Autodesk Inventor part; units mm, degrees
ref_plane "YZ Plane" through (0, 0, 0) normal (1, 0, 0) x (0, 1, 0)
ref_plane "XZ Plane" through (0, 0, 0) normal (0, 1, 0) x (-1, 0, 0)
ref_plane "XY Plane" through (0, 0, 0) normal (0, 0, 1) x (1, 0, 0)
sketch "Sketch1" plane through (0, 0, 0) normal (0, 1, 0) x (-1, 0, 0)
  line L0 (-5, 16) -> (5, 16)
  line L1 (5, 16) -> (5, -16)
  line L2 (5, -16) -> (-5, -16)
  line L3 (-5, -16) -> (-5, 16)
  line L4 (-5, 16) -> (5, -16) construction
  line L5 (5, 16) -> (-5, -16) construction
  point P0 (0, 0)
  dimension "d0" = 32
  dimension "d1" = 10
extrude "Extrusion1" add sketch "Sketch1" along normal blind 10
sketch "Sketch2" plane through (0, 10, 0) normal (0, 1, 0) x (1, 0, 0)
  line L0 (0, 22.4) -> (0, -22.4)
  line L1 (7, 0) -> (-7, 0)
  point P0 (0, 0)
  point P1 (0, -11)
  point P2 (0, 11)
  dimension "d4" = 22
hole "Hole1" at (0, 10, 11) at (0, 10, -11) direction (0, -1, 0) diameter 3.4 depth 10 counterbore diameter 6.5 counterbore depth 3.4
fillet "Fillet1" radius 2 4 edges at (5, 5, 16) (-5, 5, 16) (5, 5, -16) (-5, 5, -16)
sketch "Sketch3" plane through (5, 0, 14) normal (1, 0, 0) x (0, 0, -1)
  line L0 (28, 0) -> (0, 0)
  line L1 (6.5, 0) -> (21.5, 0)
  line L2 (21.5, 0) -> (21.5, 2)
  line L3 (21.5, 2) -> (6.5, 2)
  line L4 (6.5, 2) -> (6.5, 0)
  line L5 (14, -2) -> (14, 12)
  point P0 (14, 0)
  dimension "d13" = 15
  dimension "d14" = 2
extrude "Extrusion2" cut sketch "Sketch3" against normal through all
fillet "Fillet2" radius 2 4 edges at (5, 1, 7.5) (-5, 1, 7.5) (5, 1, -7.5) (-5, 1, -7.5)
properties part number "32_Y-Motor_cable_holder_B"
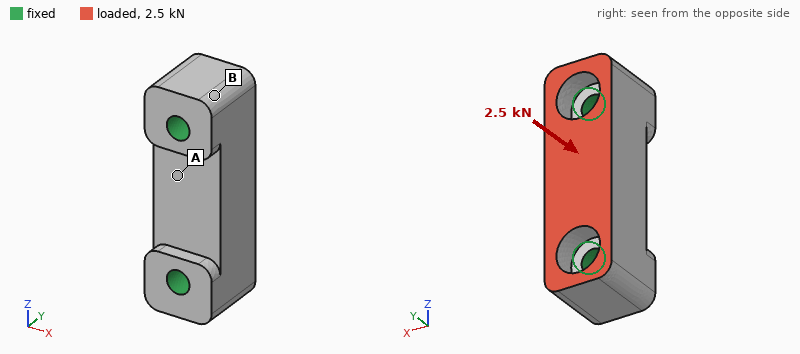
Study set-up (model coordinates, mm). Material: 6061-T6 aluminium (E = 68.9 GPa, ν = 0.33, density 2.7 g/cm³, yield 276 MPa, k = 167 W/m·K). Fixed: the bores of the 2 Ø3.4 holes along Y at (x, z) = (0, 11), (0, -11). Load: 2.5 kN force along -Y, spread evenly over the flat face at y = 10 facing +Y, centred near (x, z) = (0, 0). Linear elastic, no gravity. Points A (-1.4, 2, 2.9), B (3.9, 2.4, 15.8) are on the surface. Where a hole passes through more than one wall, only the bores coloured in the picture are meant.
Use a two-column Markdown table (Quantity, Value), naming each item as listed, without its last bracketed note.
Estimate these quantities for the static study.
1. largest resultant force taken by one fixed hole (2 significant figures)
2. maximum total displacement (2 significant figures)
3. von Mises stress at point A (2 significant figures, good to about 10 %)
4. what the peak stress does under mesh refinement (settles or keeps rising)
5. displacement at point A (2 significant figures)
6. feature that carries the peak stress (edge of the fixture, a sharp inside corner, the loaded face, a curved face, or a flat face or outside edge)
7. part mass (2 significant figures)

| Quantity | Value |
|---|---|
| largest resultant force taken by one fixed hole | 1.3 kN |
| maximum total displacement | 5.9 µm |
| von Mises stress at point A | 14 MPa |
| what the peak stress does under mesh refinement | keeps rising |
| displacement at point A | 4.7 µm |
| feature that carries the peak stress | edge of the fixture |
| part mass | 6.8 g |
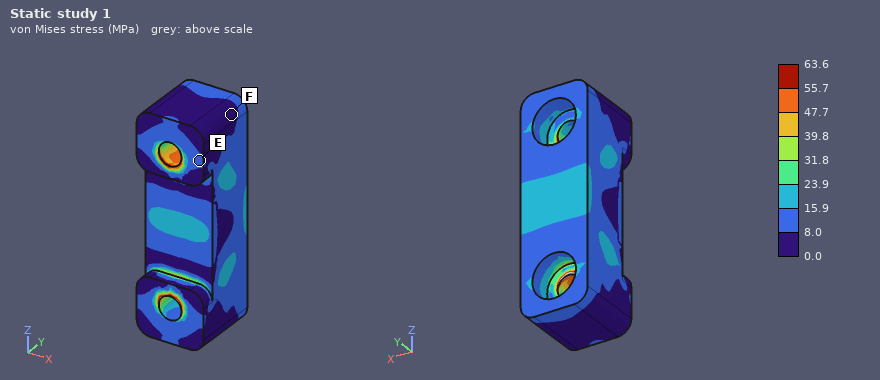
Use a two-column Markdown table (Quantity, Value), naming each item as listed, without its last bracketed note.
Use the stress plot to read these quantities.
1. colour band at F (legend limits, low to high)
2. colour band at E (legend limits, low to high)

| Quantity | Value |
|---|---|
| colour band at F | 0.0 to 8.0 MPa |
| colour band at E | 8.0 to 15.9 MPa |
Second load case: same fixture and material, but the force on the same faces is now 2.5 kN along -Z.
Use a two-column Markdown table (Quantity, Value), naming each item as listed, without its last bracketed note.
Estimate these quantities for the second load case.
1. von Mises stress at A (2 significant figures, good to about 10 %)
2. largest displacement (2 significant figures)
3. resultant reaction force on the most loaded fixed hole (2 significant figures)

| Quantity | Value |
|---|---|
| von Mises stress at A | 8.9 MPa |
| largest displacement | 7.8 µm |
| resultant reaction force on the most loaded fixed hole | 1.4 kN |
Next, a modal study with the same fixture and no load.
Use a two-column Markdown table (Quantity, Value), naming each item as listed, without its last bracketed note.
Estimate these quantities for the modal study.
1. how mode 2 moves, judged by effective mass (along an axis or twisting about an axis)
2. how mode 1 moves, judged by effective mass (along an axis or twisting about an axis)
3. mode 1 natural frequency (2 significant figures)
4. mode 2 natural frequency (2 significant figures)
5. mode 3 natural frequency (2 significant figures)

| Quantity | Value |
|---|---|
| how mode 2 moves, judged by effective mass | along Y |
| how mode 1 moves, judged by effective mass | along X |
| mode 1 natural frequency | 41 kHz |
| mode 2 natural frequency | 50 kHz |
| mode 3 natural frequency | 59 kHz |
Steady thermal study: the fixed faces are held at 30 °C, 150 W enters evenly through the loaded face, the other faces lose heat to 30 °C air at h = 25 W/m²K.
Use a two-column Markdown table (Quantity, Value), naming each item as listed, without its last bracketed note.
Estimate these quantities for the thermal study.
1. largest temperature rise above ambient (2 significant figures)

| Quantity | Value |
|---|---|
| largest temperature rise above ambient | 45 K |
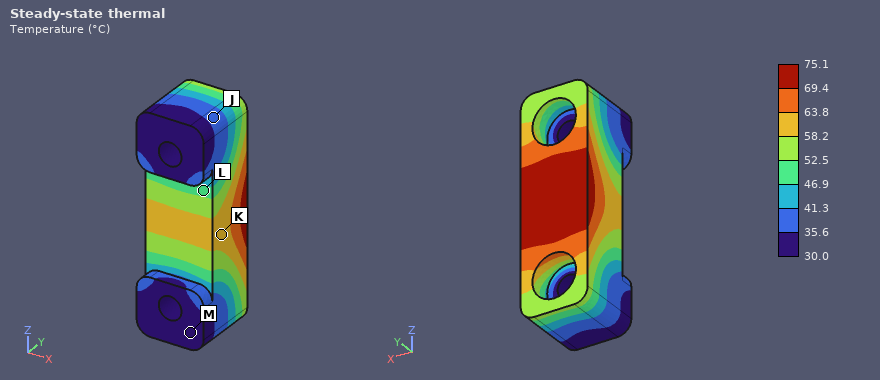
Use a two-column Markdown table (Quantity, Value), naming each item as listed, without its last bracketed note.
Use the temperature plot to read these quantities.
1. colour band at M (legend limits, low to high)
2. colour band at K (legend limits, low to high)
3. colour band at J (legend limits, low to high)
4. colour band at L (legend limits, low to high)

| Quantity | Value |
|---|---|
| colour band at M | 30.0 to 35.6 °C |
| colour band at K | 58.2 to 63.8 °C |
| colour band at J | 35.6 to 41.3 °C |
| colour band at L | 46.9 to 52.5 °C |
